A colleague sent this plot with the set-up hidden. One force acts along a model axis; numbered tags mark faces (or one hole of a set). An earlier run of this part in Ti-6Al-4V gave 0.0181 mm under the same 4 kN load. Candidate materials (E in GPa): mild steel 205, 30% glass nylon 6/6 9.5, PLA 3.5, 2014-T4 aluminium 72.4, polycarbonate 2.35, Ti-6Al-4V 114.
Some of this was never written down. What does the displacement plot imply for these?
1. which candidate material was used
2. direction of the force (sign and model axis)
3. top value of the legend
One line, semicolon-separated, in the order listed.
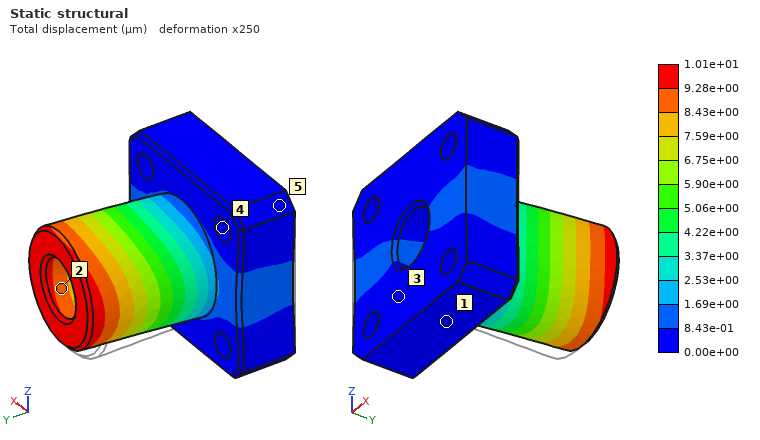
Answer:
mild steel; +X; 1.01e+01 µm
